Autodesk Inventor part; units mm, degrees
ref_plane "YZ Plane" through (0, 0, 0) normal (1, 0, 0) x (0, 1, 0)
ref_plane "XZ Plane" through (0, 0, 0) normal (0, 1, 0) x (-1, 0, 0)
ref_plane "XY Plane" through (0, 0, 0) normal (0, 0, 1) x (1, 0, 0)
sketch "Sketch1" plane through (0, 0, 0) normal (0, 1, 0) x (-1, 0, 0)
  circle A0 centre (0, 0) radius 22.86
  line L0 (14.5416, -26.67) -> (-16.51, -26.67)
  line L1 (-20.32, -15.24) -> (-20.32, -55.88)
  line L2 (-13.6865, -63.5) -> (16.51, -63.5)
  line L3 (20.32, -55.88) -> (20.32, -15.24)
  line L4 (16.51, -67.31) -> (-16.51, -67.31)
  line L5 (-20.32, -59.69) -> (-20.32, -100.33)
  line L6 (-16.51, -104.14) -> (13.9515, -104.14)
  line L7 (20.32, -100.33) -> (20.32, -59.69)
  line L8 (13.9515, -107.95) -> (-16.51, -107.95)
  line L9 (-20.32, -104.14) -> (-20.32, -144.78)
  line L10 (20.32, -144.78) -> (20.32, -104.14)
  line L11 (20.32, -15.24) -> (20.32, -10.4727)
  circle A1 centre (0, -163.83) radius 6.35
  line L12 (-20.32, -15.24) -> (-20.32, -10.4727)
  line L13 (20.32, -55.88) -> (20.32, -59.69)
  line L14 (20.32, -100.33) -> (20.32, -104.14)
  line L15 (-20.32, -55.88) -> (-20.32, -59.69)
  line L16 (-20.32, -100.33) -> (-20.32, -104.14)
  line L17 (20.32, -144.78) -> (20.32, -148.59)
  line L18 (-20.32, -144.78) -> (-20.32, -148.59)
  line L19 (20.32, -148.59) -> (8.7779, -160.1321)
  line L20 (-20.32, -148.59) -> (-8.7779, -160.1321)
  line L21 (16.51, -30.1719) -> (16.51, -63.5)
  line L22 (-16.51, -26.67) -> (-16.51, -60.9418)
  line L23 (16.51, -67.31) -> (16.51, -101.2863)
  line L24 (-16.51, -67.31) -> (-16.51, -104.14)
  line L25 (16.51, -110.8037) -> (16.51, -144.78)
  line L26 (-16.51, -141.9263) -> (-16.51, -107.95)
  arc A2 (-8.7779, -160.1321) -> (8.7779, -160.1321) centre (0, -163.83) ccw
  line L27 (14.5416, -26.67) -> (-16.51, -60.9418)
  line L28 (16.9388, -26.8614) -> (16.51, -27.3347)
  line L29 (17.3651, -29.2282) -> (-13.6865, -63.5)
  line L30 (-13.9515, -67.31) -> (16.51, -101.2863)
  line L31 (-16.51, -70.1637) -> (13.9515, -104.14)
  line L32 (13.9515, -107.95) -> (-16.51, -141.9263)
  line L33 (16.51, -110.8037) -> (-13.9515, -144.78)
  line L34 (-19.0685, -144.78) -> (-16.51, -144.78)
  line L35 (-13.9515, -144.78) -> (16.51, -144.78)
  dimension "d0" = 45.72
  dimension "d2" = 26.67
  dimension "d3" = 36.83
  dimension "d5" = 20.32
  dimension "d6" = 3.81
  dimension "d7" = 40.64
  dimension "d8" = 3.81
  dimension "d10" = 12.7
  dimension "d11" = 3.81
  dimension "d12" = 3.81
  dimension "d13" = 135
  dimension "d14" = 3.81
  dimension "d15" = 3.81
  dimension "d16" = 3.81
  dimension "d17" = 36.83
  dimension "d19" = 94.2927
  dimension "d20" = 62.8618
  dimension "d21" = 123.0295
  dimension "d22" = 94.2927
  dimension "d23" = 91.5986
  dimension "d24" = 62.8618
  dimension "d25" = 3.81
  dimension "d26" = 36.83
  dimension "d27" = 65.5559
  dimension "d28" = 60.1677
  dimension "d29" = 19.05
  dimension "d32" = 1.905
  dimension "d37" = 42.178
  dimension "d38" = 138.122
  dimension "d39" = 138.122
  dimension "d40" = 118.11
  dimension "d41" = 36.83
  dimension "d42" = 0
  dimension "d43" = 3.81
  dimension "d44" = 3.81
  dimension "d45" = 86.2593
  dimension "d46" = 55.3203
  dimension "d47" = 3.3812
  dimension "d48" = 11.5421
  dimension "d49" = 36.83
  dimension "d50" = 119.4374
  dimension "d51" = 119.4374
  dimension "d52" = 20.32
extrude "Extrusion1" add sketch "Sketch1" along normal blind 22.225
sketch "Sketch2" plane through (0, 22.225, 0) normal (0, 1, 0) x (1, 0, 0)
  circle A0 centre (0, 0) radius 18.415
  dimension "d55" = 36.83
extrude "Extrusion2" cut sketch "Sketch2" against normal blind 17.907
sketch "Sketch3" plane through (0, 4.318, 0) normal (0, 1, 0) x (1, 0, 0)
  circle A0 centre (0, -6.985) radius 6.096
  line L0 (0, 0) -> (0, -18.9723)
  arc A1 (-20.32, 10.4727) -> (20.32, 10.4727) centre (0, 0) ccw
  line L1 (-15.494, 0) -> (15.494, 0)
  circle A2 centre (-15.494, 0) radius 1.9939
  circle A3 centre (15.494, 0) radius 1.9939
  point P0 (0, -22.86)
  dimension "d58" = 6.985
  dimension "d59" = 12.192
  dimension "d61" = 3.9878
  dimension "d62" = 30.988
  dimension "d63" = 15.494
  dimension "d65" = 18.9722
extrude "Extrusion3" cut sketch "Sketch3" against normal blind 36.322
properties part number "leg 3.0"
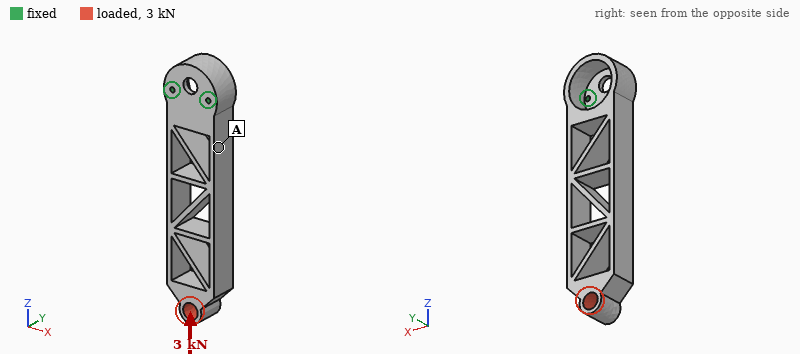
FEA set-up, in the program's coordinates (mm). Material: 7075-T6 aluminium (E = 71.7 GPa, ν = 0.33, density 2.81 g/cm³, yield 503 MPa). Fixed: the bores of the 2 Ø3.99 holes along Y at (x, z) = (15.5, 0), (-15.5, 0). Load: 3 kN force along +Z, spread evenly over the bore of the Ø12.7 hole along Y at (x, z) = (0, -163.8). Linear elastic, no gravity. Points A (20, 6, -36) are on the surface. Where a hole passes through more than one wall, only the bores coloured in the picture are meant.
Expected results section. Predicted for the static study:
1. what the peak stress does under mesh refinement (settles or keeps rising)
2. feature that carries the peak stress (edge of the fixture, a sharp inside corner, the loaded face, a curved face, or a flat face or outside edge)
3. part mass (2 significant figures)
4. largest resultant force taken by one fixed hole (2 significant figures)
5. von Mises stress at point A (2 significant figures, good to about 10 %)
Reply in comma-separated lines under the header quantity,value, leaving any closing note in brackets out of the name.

quantity,value
what the peak stress does under mesh refinement,keeps rising
feature that carries the peak stress,edge of the fixture
part mass,210 g
largest resultant force taken by one fixed hole,1.5 kN
von Mises stress at point A,16 MPa
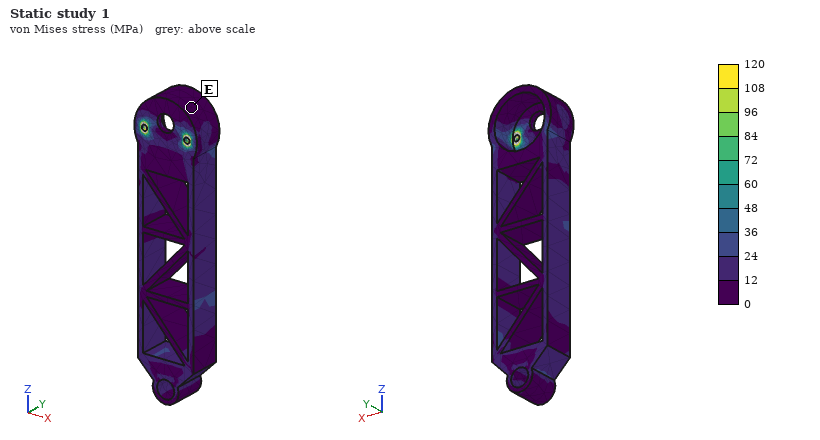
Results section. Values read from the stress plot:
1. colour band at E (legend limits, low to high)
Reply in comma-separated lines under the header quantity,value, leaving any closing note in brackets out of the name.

quantity,value
colour band at E,0 to 12 MPa
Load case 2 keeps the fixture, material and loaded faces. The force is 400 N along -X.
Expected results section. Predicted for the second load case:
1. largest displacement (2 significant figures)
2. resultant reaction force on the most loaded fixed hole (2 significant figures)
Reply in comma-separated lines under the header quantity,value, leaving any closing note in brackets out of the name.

quantity,value
largest displacement,0.23 mm
resultant reaction force on the most loaded fixed hole,2.0 kN
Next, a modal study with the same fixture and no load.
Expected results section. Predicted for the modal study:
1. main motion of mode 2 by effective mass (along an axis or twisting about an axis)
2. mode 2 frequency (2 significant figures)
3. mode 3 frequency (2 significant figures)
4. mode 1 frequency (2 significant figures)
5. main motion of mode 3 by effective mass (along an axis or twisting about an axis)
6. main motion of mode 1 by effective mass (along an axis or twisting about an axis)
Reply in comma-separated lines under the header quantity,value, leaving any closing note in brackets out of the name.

quantity,value
main motion of mode 2 by effective mass,along X
mode 2 frequency,940 Hz
mode 3 frequency,2000 Hz
mode 1 frequency,280 Hz
main motion of mode 3 by effective mass,twisting about Z
main motion of mode 1 by effective mass,along Y
